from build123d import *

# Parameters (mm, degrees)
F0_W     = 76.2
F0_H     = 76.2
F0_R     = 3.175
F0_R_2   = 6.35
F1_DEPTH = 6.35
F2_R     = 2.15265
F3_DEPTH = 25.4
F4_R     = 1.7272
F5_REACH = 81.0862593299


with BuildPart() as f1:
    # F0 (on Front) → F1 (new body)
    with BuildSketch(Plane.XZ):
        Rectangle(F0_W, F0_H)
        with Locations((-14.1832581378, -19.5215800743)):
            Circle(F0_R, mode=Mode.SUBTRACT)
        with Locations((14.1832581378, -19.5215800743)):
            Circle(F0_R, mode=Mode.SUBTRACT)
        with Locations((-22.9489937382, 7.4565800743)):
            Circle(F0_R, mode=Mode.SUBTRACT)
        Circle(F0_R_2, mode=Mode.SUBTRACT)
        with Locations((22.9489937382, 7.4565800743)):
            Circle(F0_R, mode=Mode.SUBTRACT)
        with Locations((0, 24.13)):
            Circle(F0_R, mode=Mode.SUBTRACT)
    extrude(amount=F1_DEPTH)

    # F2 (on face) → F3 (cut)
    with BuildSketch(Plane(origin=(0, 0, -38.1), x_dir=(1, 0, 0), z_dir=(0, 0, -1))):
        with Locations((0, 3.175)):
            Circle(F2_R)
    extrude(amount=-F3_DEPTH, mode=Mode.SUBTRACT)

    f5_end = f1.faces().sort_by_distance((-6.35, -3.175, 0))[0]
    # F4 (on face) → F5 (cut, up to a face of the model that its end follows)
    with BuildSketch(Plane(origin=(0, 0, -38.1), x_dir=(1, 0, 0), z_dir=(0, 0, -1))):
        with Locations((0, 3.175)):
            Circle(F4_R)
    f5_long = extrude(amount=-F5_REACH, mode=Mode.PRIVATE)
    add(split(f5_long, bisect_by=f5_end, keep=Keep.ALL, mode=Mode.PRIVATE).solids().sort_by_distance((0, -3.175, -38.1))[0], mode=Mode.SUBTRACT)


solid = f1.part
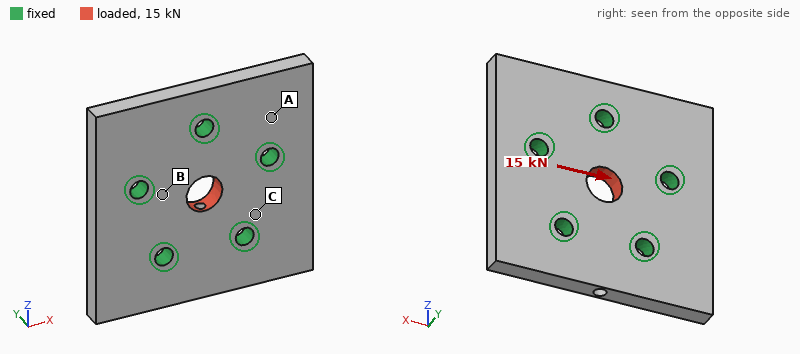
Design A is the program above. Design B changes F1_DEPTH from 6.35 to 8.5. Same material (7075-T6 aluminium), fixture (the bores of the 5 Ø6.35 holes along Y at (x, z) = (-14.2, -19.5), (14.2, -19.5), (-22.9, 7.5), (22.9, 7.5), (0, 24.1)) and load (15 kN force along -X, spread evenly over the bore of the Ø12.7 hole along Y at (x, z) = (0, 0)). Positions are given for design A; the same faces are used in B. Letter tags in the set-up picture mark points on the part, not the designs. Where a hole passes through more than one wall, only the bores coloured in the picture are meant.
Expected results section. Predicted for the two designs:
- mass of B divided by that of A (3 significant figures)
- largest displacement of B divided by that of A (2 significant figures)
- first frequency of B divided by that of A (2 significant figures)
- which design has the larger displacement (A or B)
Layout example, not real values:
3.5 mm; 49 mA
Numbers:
1.34; 0.74; 1.3; A
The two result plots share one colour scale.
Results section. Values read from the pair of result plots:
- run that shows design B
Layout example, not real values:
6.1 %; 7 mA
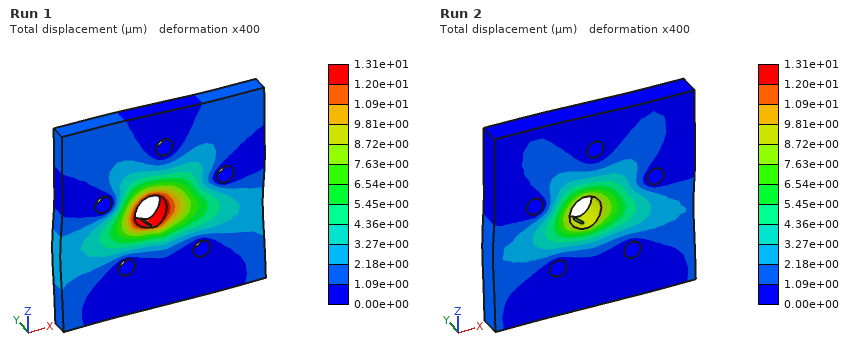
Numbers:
Run 2
